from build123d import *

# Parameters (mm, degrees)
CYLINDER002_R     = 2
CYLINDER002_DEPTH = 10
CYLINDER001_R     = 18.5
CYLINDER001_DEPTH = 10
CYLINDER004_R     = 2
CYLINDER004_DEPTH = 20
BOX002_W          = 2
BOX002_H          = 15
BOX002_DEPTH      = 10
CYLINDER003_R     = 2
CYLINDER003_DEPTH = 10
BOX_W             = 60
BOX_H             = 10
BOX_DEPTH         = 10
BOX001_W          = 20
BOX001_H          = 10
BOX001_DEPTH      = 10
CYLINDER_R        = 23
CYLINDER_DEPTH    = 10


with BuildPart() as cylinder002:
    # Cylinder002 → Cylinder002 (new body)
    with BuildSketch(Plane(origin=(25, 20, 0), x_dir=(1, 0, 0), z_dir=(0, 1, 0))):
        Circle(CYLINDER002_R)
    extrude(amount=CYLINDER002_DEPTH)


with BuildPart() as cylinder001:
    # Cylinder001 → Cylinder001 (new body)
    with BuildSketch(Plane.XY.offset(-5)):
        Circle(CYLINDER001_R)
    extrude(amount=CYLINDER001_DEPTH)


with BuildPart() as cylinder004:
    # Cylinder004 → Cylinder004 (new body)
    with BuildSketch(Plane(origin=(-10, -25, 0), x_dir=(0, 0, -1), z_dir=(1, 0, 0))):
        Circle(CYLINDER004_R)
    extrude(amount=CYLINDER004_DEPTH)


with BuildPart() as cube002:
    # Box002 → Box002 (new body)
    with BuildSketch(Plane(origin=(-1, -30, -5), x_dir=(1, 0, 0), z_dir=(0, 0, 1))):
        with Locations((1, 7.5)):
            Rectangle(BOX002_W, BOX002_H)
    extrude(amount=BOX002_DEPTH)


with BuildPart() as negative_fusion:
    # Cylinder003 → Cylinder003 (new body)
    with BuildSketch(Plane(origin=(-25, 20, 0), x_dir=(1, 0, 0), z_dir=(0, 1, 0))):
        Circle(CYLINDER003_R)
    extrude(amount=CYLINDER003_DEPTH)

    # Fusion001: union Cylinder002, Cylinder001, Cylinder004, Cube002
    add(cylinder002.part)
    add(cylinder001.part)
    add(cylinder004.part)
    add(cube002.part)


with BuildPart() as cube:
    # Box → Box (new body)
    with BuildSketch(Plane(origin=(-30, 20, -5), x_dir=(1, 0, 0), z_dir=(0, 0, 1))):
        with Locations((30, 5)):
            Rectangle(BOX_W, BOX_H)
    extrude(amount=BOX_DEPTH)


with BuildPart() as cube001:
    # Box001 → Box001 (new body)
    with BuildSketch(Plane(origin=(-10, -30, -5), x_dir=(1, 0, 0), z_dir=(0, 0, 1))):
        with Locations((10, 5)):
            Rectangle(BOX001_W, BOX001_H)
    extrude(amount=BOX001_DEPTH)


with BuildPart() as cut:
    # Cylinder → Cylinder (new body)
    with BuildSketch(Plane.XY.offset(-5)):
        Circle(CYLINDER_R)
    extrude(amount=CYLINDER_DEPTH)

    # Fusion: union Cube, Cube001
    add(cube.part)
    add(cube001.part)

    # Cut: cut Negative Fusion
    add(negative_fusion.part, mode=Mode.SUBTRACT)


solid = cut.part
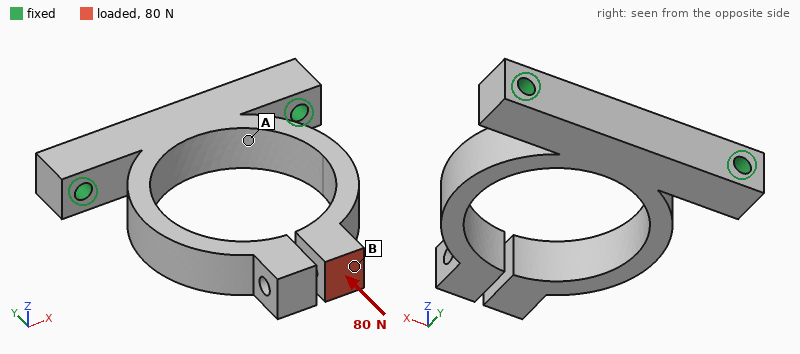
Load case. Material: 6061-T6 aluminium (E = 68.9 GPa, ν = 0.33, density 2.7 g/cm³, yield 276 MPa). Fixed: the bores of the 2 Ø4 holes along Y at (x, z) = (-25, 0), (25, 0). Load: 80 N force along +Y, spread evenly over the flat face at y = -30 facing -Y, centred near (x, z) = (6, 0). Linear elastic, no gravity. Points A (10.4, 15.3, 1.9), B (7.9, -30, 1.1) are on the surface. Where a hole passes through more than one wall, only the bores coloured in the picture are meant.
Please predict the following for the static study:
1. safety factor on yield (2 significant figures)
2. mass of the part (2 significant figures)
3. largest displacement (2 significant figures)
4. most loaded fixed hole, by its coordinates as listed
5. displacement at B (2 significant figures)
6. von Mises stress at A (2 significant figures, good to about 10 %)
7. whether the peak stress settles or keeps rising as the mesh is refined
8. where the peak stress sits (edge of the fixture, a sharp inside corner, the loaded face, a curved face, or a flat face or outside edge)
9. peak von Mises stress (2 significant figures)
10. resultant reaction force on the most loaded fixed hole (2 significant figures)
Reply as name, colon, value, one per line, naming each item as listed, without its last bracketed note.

safety factor on yield: 6.7
mass of the part: 33 g
largest displacement: 0.28 mm
most loaded fixed hole, by its coordinates as listed: (25, 0)
displacement at B: 0.25 mm
von Mises stress at A: 16 MPa
whether the peak stress settles or keeps rising as the mesh is refined: settles
where the peak stress sits: a curved face
peak von Mises stress: 41 MPa
resultant reaction force on the most loaded fixed hole: 54 N
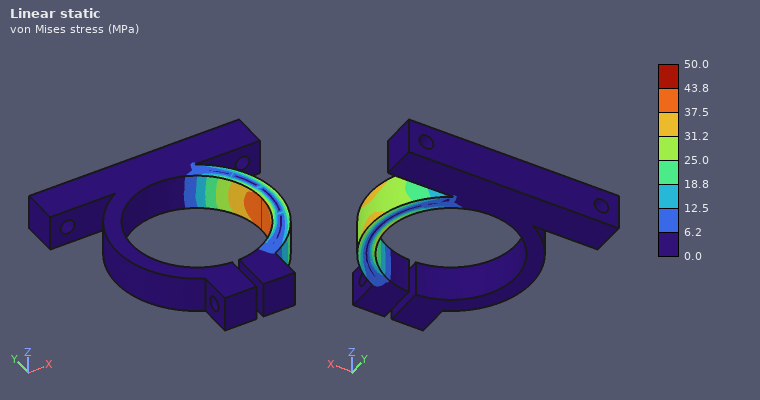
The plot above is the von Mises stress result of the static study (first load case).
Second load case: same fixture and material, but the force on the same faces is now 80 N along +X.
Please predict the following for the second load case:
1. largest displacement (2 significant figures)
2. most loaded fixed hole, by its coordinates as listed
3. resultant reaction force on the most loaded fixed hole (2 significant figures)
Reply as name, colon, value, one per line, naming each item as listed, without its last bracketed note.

largest displacement: 0.86 mm
most loaded fixed hole, by its coordinates as listed: (-25, 0)
resultant reaction force on the most loaded fixed hole: 170 N
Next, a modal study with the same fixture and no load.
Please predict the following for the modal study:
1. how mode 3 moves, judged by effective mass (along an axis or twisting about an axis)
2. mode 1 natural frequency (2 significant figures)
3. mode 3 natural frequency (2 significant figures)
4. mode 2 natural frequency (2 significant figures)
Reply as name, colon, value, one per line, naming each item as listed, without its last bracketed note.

how mode 3 moves, judged by effective mass: along Z
mode 1 natural frequency: 960 Hz
mode 3 natural frequency: 1200 Hz
mode 2 natural frequency: 960 Hz
